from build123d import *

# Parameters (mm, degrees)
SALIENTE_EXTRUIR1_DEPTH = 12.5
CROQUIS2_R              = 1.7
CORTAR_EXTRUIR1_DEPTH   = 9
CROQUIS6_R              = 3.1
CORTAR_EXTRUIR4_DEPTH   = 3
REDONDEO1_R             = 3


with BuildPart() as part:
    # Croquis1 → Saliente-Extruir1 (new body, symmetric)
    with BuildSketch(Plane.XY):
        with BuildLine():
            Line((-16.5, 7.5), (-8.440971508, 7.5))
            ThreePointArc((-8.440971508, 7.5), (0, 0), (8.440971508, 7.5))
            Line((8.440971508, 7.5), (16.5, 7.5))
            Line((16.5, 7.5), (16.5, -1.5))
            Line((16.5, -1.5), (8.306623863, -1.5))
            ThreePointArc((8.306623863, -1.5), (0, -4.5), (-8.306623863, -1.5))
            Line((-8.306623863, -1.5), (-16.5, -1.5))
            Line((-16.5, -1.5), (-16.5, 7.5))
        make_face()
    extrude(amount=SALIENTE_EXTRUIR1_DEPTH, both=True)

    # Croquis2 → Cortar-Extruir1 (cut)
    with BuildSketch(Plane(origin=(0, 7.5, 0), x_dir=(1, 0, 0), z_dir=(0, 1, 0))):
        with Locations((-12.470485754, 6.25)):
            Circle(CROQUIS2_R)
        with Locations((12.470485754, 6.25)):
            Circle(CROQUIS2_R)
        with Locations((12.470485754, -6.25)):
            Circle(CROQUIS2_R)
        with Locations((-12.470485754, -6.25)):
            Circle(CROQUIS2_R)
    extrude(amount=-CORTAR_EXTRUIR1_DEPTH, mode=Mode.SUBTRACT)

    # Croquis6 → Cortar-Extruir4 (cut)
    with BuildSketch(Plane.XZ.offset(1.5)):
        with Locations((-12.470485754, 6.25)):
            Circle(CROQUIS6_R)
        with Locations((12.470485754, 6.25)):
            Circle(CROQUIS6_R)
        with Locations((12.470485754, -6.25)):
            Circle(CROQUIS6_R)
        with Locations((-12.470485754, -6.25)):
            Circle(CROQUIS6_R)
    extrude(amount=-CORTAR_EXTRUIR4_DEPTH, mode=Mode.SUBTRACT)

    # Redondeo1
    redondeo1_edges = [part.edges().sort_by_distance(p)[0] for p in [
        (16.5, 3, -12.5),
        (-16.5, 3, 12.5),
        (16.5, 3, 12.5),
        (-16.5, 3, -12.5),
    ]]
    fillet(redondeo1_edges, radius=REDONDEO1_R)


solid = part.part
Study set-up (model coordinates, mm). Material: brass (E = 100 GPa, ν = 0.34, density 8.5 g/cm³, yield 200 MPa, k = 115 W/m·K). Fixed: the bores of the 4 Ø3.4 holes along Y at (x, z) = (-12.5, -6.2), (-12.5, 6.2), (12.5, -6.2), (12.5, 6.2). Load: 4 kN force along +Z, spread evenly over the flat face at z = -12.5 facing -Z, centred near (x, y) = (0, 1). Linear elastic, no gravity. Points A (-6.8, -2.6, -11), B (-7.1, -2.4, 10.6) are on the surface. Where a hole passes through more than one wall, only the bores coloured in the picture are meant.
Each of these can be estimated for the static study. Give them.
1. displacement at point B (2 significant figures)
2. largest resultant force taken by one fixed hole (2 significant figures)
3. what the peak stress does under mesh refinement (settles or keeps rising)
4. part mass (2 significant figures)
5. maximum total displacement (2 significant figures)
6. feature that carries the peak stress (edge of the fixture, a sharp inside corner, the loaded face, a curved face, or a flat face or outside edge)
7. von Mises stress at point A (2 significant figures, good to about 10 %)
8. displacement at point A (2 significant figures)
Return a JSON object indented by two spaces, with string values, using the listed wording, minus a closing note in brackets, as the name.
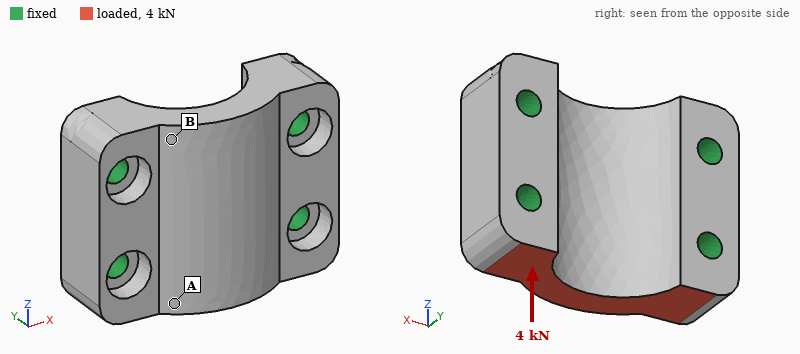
{
  "displacement at point B": "2.6 µm",
  "largest resultant force taken by one fixed hole": "1.5 kN",
  "what the peak stress does under mesh refinement": "keeps rising",
  "part mass": "44 g",
  "maximum total displacement": "8.2 µm",
  "feature that carries the peak stress": "edge of the fixture",
  "von Mises stress at point A": "21 MPa",
  "displacement at point A": "5.8 µm"
}
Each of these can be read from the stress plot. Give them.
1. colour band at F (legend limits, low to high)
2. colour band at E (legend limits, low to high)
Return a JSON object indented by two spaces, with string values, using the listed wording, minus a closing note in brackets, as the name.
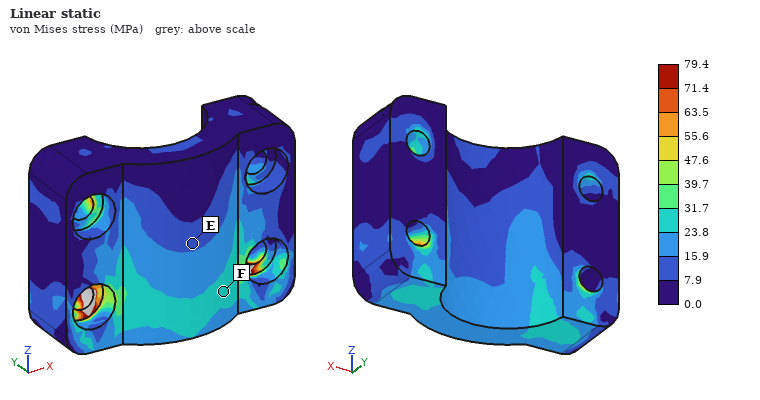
{
  "colour band at F": "23.8 to 31.7 MPa",
  "colour band at E": "7.9 to 15.9 MPa"
}
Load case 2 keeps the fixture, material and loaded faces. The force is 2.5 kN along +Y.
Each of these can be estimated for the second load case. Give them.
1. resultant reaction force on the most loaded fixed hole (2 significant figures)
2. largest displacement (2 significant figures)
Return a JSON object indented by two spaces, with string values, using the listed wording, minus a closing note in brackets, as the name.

{
  "resultant reaction force on the most loaded fixed hole": "1.6 kN",
  "largest displacement": "14 µm"
}
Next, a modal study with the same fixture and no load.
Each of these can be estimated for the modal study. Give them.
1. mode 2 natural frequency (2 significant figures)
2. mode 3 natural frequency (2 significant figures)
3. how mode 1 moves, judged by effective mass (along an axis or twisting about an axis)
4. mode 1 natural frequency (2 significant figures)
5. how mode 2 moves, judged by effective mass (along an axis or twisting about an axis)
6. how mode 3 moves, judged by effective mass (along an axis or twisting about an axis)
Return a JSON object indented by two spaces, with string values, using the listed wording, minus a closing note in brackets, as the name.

{
  "mode 2 natural frequency": "33 kHz",
  "mode 3 natural frequency": "37 kHz",
  "how mode 1 moves, judged by effective mass": "along Z",
  "mode 1 natural frequency": "27 kHz",
  "how mode 2 moves, judged by effective mass": "along Y",
  "how mode 3 moves, judged by effective mass": "along X"
}
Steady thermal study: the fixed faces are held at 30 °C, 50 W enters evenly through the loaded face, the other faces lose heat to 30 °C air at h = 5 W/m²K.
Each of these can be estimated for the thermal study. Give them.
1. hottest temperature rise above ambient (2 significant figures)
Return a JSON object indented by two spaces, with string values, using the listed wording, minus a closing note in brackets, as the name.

{
  "hottest temperature rise above ambient": "26 K"
}
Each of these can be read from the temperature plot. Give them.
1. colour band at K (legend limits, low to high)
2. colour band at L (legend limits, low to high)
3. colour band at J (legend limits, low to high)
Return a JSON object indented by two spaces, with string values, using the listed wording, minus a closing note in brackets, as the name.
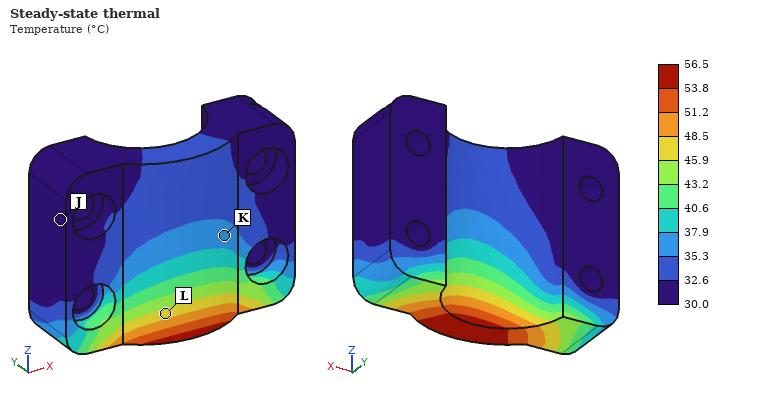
{
  "colour band at K": "35.3 to 37.9 °C",
  "colour band at L": "45.9 to 48.5 °C",
  "colour band at J": "30.0 to 32.6 °C"
}
